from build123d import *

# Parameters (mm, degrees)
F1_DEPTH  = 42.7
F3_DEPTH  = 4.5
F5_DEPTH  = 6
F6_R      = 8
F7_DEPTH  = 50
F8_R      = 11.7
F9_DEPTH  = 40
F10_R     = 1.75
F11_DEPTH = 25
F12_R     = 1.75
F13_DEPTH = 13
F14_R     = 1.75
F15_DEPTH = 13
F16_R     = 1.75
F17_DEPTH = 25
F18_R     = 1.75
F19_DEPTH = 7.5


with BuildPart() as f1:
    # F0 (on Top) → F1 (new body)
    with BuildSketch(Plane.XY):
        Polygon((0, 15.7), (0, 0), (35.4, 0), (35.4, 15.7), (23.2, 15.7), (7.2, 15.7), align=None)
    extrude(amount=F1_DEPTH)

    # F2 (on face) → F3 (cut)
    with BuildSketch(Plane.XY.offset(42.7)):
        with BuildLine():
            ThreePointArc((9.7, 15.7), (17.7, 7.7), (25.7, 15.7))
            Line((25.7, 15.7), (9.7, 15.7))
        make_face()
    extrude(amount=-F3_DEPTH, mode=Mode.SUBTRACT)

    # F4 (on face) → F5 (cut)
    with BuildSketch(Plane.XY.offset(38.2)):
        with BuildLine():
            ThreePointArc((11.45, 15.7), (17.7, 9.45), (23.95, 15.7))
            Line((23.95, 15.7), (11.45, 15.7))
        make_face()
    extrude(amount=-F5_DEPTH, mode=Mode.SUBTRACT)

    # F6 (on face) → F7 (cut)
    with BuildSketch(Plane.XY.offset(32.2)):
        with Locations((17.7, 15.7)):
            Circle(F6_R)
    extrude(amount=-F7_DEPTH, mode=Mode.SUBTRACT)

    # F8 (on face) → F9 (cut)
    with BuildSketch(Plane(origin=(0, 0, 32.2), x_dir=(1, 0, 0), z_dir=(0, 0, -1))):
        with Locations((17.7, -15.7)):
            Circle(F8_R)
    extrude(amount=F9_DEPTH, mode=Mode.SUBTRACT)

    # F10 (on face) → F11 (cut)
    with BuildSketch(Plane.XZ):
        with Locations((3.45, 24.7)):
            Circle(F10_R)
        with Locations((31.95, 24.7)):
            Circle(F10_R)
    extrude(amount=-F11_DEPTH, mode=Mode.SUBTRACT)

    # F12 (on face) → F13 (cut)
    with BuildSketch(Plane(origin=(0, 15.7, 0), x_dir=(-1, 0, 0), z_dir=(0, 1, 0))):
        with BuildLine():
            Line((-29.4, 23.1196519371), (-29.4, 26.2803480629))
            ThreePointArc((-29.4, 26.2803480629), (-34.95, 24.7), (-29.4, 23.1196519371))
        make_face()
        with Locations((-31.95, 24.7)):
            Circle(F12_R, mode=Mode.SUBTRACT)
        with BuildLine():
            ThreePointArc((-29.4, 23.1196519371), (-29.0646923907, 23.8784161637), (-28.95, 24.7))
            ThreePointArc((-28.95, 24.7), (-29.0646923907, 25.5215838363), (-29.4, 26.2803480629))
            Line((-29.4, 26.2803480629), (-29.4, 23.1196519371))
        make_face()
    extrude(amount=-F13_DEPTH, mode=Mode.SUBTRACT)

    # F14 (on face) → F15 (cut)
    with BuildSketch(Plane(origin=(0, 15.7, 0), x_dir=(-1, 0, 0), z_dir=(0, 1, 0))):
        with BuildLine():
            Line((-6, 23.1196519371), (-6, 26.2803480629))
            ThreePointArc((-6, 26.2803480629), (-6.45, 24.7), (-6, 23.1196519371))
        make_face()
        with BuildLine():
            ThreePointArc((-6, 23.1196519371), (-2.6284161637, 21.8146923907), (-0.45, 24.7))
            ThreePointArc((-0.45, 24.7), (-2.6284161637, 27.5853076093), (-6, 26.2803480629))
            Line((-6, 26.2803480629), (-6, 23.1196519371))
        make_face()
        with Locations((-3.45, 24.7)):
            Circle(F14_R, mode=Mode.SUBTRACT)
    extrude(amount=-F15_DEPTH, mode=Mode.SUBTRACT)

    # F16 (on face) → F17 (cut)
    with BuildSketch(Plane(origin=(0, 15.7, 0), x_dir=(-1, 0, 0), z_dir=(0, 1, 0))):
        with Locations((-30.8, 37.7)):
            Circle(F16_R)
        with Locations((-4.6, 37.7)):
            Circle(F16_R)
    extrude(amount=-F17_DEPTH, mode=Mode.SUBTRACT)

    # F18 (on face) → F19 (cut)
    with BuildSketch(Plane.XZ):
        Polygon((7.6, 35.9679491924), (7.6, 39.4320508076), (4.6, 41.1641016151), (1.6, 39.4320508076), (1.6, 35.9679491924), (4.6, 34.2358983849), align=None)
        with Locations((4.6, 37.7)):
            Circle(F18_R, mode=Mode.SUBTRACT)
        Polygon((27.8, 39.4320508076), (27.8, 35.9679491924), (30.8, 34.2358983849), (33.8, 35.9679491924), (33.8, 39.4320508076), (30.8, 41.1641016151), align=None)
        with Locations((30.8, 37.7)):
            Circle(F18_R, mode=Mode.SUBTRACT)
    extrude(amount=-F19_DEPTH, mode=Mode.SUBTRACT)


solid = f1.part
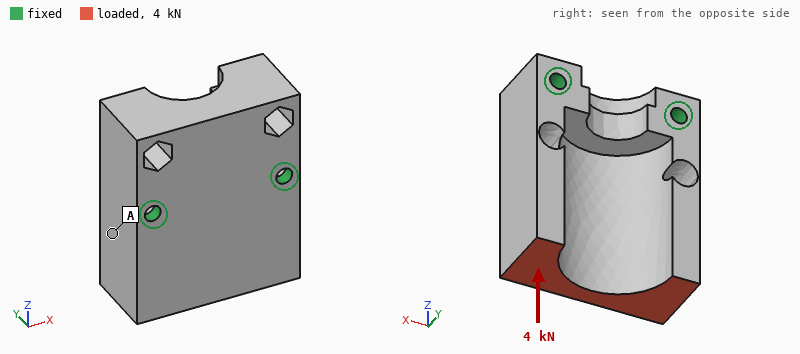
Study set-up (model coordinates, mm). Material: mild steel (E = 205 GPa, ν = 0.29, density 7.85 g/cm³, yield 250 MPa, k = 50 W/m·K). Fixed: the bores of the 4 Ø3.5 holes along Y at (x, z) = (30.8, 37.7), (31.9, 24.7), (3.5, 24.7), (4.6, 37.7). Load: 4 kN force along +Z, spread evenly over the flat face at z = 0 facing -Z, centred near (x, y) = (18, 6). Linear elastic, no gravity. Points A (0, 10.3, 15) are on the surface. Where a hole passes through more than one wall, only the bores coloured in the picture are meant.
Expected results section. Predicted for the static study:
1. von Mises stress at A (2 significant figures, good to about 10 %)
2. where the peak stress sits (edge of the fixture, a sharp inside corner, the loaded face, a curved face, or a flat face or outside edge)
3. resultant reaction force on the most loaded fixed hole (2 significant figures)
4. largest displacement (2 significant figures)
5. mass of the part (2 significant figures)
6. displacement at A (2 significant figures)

14 MPa
a curved face
1.0 kN
8.5 µm
110 g
4.0 µm
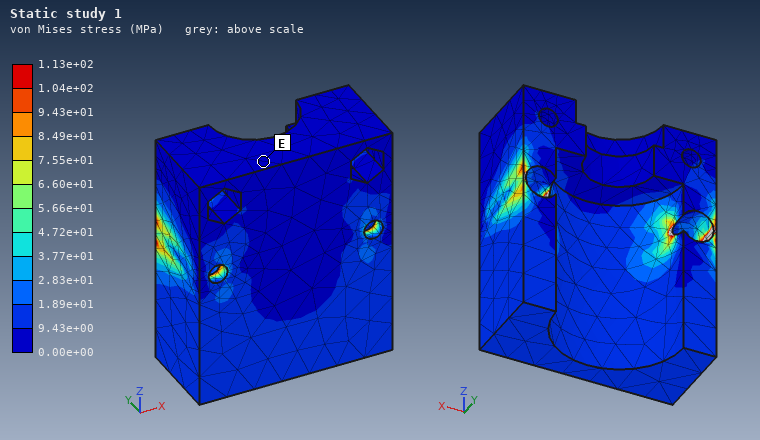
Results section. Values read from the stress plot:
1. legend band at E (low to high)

0.00e+00 to 9.43e+00 MPa
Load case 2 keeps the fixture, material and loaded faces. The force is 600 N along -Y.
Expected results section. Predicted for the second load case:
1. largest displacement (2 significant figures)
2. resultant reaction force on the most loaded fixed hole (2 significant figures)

11 µm
660 N
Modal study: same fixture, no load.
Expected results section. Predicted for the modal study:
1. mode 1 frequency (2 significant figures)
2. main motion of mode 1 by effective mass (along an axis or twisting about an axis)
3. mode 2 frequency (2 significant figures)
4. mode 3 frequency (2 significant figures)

8100 Hz
along Y
11 kHz
15 kHz
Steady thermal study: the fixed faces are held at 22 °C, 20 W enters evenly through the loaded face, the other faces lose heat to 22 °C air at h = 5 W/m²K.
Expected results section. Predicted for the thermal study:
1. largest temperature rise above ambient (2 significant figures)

40 K
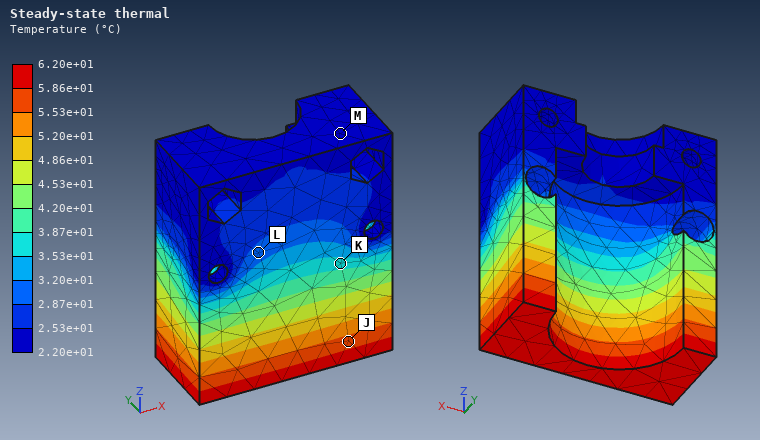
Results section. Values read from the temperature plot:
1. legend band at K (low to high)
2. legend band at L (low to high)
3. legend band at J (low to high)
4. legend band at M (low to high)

3.53e+01 to 3.87e+01 °C
2.87e+01 to 3.20e+01 °C
5.53e+01 to 5.86e+01 °C
2.20e+01 to 2.53e+01 °C
